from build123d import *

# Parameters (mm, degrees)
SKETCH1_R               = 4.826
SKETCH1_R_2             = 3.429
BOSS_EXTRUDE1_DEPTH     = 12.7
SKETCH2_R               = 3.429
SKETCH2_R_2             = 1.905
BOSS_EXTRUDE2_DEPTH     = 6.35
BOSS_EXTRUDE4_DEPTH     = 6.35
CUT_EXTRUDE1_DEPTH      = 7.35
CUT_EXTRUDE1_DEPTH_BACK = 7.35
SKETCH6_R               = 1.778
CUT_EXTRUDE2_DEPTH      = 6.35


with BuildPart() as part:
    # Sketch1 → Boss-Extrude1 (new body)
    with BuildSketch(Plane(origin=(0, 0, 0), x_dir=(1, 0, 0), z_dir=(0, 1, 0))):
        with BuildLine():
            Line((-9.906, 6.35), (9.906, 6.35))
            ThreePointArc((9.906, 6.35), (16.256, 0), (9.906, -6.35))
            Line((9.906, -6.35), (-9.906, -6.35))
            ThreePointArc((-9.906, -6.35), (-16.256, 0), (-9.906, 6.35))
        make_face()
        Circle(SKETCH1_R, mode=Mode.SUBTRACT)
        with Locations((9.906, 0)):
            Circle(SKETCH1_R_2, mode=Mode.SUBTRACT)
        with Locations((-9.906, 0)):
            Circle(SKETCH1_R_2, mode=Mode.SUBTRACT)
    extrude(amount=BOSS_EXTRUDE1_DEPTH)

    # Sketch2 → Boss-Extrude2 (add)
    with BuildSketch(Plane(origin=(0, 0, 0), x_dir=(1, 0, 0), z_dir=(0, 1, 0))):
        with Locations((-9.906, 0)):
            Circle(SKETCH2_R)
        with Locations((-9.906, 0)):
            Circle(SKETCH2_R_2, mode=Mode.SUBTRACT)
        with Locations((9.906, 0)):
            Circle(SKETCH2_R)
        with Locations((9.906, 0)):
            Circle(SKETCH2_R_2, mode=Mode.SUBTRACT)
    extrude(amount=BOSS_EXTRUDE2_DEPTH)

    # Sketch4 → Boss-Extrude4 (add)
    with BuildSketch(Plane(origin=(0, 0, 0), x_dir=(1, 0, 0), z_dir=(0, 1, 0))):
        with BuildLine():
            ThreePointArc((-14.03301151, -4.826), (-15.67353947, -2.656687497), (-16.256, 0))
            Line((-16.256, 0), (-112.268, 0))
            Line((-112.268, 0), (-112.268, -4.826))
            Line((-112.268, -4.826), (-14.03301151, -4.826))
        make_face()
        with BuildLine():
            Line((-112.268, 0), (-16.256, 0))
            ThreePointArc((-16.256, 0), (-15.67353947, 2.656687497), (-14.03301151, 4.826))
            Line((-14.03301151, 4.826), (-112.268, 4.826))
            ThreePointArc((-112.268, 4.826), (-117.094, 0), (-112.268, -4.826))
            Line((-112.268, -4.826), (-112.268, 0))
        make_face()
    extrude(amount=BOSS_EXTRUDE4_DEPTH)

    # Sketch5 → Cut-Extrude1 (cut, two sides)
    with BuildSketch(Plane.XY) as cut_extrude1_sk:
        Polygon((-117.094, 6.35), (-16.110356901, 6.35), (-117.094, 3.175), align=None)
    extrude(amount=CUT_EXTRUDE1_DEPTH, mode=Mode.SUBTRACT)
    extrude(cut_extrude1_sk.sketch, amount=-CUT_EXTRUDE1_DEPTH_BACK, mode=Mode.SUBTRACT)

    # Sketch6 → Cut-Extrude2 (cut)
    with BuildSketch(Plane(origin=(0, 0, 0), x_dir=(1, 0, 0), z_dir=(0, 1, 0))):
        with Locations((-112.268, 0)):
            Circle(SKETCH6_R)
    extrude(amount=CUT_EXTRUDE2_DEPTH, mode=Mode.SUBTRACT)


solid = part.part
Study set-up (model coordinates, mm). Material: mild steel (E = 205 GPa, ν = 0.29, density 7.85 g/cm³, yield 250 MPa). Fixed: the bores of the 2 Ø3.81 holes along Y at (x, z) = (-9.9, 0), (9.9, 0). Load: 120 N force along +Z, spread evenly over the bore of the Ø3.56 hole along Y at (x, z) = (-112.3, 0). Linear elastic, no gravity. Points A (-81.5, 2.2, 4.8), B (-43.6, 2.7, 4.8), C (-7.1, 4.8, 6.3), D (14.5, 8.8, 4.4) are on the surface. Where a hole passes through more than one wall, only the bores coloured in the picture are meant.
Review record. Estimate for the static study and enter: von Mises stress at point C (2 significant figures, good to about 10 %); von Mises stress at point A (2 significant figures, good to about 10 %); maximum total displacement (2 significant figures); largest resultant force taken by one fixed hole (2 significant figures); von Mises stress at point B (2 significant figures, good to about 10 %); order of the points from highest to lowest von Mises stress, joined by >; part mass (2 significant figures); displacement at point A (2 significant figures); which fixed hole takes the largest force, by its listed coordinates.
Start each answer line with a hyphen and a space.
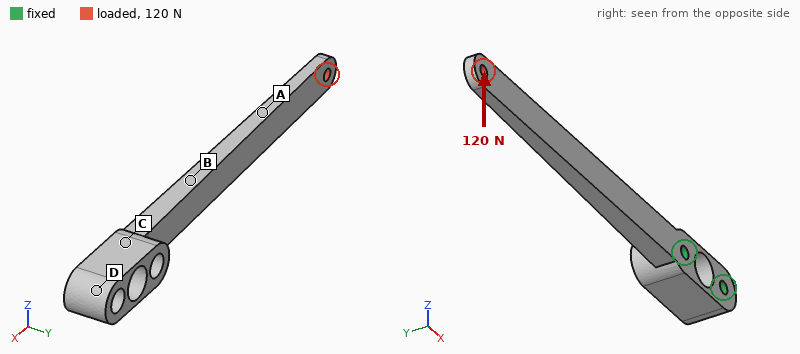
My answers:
- 23 MPa
- 55 MPa
- 0.54 mm
- 280 N
- 97 MPa
- B > A > C > D
- 62 g
- 0.27 mm
- (-9.9, 0)
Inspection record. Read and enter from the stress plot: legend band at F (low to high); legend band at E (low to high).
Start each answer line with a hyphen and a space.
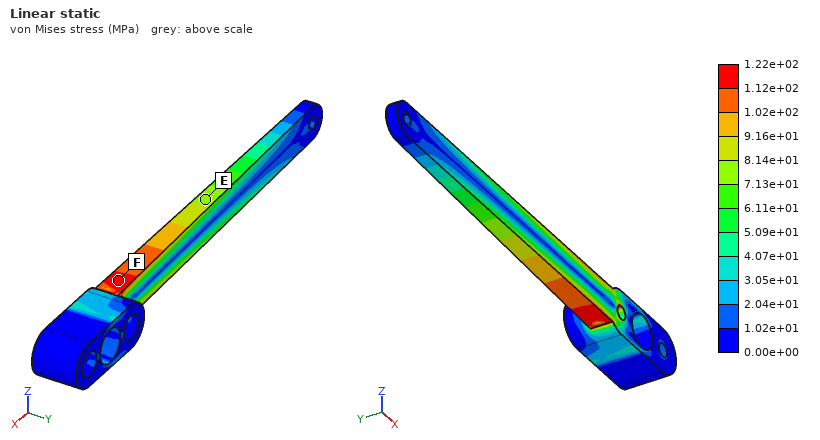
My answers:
- 1.12e+02 to 1.22e+02 MPa
- 7.13e+01 to 8.14e+01 MPa
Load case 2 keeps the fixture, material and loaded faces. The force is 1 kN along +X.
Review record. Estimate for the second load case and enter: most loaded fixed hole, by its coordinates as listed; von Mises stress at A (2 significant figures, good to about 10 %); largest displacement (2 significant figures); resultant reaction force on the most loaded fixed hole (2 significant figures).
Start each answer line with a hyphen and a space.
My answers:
- (-9.9, 0)
- 24 MPa
- 0.21 mm
- 970 N
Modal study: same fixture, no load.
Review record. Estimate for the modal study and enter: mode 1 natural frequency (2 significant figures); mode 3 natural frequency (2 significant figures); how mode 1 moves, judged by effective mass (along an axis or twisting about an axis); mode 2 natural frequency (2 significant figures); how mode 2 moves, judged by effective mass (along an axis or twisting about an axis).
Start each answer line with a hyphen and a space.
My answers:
- 550 Hz
- 2600 Hz
- along Y
- 880 Hz
- along Z
